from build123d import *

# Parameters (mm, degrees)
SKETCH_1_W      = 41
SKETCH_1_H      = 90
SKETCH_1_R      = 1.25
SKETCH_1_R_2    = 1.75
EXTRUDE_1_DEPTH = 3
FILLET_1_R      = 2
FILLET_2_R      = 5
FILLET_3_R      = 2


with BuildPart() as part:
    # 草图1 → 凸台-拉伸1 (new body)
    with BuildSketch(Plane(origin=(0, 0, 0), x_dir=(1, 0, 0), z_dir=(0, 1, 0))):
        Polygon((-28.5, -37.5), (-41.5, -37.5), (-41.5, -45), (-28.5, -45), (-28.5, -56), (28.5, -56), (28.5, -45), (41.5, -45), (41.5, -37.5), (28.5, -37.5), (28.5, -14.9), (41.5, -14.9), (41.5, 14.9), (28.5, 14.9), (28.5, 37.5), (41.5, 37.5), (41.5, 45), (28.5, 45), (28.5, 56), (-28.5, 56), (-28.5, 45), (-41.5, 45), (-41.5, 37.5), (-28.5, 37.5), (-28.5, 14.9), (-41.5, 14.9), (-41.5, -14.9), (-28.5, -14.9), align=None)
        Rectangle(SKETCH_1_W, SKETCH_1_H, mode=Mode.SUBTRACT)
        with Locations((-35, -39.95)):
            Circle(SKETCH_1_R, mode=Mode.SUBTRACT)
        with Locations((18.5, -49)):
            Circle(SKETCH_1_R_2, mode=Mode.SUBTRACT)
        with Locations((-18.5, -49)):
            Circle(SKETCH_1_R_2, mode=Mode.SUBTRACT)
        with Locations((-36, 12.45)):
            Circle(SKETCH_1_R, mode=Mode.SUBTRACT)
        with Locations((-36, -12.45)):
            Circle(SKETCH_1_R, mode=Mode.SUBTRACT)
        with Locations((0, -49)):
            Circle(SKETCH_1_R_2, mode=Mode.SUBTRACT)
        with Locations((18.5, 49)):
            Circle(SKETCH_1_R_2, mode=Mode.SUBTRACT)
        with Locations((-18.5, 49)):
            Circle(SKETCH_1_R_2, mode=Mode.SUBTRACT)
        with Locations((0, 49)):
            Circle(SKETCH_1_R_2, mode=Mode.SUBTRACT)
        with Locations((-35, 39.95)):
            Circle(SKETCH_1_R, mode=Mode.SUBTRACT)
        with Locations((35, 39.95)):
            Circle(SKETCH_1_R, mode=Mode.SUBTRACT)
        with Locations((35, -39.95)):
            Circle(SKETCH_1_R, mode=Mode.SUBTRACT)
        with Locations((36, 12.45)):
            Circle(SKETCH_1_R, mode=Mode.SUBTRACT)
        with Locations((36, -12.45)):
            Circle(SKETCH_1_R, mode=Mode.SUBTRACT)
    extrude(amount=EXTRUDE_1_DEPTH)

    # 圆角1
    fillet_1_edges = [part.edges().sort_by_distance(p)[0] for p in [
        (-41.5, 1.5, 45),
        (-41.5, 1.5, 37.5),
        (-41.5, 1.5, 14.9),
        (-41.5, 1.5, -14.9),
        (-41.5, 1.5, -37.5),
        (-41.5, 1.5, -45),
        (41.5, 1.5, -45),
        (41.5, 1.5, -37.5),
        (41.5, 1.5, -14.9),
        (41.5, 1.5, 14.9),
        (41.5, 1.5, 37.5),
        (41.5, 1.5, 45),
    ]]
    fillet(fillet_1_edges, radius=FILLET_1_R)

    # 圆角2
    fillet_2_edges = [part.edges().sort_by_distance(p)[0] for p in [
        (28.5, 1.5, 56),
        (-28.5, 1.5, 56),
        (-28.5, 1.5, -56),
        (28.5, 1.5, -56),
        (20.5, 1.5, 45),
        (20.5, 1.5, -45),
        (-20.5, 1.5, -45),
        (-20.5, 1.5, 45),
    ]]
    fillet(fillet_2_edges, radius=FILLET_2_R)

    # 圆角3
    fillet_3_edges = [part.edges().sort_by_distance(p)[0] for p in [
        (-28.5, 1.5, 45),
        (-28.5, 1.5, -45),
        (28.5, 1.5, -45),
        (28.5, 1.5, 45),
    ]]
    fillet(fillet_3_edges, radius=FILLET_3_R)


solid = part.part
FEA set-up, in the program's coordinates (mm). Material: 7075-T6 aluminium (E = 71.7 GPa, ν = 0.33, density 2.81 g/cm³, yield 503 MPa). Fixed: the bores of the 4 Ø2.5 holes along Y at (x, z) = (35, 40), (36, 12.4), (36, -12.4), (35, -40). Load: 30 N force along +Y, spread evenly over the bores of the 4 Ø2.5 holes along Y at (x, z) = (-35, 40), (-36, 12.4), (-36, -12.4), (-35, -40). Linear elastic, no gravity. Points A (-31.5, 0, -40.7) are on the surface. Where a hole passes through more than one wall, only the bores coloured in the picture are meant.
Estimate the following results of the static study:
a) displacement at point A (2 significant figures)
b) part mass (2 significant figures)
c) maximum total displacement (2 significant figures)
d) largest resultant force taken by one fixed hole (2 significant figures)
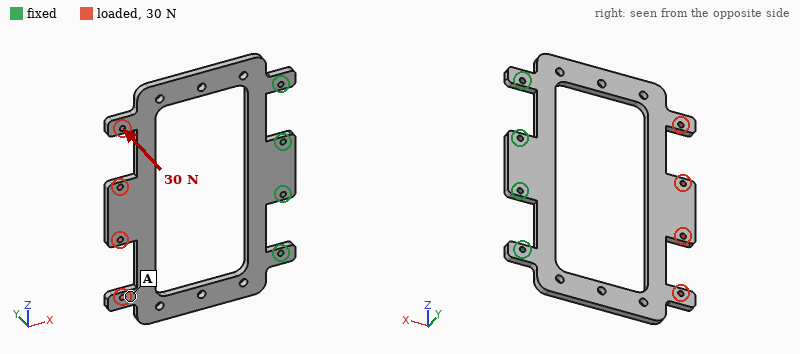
1.1 mm
32 g
1.4 mm
13 N
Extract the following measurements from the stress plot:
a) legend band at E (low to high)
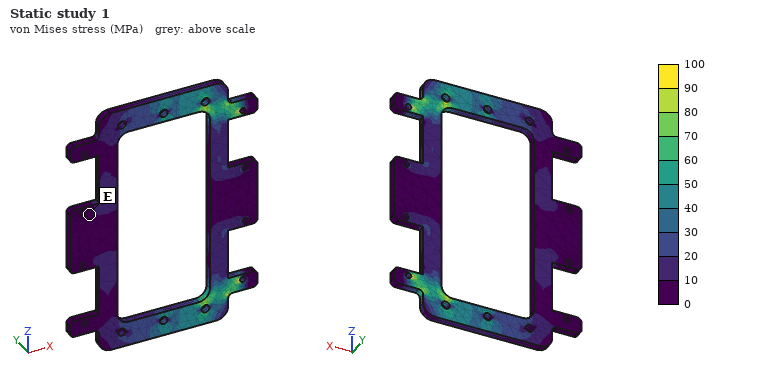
0 to 10 MPa
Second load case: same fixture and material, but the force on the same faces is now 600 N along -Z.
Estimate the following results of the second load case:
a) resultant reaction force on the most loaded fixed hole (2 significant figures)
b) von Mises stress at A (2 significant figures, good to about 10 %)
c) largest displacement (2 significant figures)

810 N
26 MPa
0.66 mm
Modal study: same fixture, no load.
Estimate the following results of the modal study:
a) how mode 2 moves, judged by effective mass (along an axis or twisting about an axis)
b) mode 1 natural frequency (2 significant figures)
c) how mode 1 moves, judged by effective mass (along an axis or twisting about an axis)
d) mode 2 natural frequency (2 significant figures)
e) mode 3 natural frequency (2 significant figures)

twisting about X
250 Hz
along Y
560 Hz
1200 Hz
